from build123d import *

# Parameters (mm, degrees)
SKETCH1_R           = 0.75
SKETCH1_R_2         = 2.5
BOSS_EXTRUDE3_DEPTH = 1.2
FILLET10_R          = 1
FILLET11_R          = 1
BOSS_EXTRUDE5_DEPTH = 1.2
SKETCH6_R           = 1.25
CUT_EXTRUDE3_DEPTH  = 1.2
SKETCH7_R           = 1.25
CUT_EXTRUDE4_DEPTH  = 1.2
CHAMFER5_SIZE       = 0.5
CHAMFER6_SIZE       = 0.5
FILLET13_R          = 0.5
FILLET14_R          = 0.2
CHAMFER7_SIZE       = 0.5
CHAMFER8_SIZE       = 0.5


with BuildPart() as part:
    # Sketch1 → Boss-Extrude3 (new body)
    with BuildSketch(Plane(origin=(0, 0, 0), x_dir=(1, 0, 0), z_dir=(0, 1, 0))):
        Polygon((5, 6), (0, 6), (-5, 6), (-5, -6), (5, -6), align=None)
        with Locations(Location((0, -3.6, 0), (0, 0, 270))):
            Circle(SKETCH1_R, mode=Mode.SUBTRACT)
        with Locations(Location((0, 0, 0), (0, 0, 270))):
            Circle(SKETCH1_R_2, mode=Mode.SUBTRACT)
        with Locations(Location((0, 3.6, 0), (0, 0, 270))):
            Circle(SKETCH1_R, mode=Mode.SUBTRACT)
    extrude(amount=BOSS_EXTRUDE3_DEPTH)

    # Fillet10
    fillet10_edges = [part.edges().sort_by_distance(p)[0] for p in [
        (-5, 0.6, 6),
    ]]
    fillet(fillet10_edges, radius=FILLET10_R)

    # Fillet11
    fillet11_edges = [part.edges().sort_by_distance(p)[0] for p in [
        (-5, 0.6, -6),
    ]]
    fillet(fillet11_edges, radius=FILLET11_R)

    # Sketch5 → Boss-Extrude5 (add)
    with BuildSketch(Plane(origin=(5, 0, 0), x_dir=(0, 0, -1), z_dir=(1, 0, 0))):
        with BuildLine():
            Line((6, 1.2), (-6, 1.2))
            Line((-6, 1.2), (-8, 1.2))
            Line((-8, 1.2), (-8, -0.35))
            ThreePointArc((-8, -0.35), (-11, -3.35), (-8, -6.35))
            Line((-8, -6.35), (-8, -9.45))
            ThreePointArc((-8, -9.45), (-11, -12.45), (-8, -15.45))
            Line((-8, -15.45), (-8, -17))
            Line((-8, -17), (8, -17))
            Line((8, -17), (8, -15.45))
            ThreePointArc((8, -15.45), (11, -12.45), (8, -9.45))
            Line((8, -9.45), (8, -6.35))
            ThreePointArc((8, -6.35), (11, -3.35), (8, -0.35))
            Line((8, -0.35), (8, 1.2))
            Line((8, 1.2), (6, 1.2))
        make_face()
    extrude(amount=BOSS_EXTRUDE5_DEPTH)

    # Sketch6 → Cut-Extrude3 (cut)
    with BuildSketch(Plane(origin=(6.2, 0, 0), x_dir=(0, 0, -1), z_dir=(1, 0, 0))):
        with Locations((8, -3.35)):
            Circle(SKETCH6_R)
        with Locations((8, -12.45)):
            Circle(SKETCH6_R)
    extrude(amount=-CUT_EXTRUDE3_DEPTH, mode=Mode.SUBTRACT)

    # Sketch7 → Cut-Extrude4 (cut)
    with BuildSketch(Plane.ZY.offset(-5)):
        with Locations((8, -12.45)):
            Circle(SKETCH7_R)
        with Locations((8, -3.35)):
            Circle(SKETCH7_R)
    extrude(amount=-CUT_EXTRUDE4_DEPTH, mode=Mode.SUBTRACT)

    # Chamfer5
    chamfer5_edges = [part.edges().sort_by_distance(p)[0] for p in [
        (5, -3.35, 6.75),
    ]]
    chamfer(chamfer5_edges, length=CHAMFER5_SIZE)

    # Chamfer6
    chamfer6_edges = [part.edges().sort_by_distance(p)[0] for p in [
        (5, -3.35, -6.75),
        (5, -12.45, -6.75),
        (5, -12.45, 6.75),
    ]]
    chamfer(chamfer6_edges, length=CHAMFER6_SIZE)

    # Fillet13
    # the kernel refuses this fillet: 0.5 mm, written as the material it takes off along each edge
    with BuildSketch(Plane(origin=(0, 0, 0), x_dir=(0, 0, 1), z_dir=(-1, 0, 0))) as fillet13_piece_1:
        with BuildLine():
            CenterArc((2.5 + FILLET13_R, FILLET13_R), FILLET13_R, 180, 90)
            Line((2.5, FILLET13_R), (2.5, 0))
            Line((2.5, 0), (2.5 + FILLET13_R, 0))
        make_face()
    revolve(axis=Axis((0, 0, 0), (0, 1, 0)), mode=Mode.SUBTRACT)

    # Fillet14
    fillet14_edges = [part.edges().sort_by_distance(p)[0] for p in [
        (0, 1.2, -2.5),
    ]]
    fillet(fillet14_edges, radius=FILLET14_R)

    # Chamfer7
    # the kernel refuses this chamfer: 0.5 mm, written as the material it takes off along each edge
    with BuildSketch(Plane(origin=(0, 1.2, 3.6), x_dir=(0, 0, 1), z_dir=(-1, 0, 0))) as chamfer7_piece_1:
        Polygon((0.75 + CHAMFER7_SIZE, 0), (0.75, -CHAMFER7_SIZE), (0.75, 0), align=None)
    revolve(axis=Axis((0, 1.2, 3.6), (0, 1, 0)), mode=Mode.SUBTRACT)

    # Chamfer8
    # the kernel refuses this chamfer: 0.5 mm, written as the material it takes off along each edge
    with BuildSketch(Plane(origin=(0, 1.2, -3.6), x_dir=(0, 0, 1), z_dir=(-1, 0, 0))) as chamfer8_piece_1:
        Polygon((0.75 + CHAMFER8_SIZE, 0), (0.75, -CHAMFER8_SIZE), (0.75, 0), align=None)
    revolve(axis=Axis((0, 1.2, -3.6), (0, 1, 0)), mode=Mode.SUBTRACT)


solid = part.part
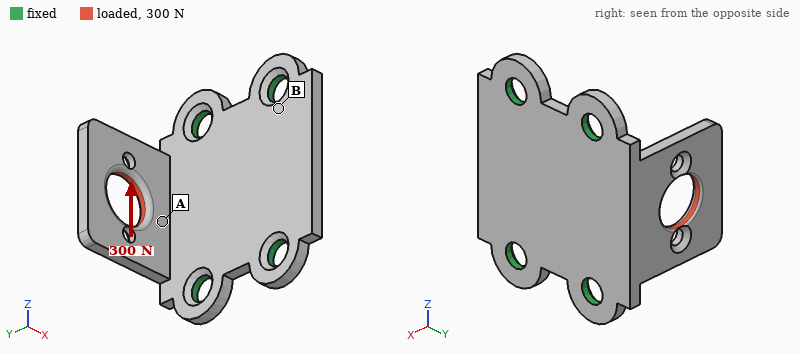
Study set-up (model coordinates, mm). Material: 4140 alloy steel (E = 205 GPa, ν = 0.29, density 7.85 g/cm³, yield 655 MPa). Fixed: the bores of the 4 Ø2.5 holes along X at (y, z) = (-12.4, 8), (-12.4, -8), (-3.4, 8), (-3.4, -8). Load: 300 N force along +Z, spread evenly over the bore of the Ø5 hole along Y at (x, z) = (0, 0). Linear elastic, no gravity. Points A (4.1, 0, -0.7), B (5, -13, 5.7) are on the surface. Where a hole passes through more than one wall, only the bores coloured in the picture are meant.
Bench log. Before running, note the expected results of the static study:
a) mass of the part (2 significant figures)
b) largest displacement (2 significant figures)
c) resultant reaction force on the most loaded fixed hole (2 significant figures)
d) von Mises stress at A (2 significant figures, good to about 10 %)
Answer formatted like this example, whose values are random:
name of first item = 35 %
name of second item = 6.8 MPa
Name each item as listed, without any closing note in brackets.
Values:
mass of the part = 3.9 g
largest displacement = 29 µm
resultant reaction force on the most loaded fixed hole = 210 N
von Mises stress at A = 100 MPa
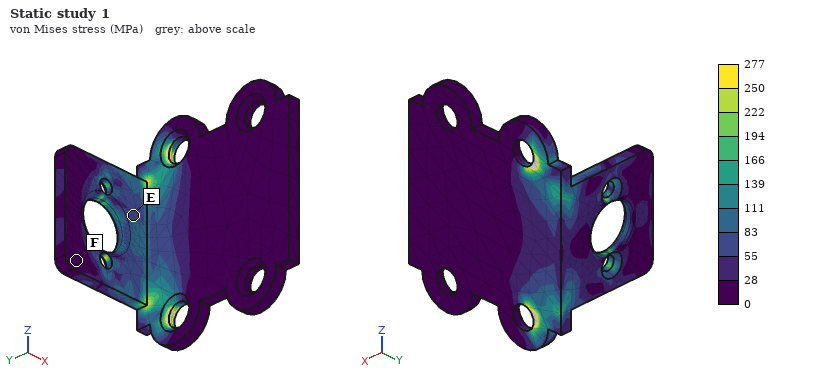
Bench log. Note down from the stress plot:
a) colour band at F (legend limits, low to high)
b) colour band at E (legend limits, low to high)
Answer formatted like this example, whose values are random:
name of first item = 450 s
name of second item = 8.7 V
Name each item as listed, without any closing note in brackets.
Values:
colour band at F = 0 to 28 MPa
colour band at E = 55 to 83 MPa
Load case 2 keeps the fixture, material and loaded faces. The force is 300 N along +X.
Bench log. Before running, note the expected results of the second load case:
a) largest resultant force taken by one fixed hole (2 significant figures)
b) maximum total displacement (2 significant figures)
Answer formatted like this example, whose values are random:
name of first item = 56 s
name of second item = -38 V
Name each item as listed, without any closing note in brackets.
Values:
largest resultant force taken by one fixed hole = 200 N
maximum total displacement = 74 µm
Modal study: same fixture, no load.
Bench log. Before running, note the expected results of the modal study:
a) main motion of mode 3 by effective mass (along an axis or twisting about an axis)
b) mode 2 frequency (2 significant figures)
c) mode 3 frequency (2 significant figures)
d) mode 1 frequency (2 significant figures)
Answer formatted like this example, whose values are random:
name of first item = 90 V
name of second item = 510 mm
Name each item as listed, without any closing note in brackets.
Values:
main motion of mode 3 by effective mass = along X
mode 2 frequency = 15 kHz
mode 3 frequency = 19 kHz
mode 1 frequency = 6000 Hz
